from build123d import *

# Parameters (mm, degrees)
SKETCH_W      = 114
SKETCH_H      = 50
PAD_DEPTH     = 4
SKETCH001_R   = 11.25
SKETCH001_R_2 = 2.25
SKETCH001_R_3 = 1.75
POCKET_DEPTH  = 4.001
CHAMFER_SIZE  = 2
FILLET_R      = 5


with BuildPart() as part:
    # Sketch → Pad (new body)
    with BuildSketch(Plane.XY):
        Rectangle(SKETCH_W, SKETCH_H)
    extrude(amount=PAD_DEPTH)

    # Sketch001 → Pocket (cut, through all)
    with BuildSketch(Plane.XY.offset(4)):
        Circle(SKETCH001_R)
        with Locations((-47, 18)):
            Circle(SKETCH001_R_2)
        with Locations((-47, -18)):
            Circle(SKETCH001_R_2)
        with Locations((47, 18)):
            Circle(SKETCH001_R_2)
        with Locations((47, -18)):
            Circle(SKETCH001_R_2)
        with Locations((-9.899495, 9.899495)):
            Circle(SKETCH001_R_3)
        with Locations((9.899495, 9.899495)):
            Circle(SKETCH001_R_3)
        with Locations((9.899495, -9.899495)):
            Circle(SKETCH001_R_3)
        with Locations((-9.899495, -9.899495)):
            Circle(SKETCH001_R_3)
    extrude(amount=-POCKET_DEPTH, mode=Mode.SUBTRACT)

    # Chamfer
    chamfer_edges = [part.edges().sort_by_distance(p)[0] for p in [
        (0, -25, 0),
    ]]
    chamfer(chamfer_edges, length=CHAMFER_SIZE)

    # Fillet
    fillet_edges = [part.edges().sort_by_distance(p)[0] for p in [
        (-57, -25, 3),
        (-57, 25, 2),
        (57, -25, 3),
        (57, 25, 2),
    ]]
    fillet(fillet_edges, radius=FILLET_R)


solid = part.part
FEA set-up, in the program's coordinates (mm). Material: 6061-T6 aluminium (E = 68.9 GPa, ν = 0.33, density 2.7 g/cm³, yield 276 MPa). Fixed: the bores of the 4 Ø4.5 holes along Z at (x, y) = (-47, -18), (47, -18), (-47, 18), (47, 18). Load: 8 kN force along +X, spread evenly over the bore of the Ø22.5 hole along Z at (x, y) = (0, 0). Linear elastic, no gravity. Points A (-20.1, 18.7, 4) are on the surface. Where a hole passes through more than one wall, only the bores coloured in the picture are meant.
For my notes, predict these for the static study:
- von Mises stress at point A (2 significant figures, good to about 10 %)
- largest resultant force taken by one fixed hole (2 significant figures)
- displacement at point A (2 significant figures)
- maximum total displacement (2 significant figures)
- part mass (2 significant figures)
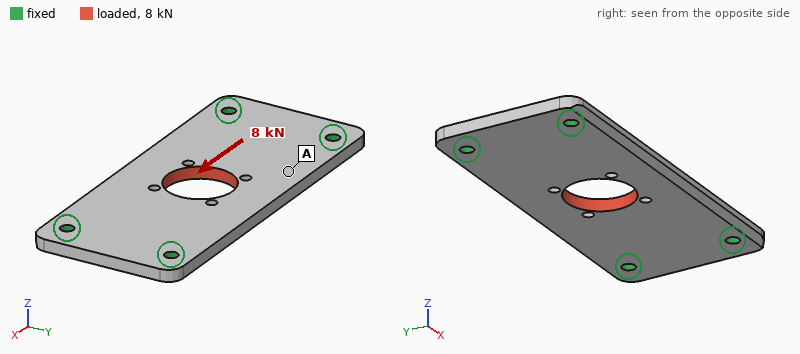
19 MPa
2.0 kN
9.8 µm
20 µm
55 g
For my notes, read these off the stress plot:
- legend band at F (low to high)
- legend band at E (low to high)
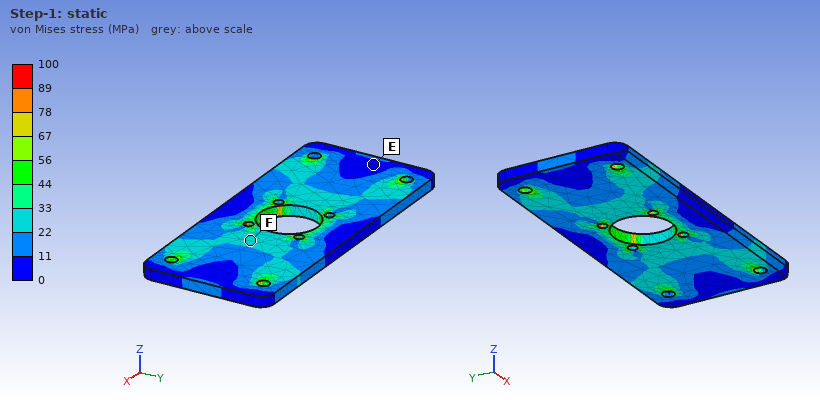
22 to 33 MPa
0 to 11 MPa
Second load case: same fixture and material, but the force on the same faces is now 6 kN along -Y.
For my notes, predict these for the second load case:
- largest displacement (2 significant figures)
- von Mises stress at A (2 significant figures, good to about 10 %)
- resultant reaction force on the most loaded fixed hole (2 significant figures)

43 µm
19 MPa
2.3 kN
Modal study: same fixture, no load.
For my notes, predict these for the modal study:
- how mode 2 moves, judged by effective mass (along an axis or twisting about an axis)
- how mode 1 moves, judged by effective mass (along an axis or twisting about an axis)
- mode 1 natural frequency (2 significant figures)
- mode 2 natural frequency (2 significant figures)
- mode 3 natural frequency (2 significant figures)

twisting about X
along Z
2300 Hz
3700 Hz
5800 Hz
